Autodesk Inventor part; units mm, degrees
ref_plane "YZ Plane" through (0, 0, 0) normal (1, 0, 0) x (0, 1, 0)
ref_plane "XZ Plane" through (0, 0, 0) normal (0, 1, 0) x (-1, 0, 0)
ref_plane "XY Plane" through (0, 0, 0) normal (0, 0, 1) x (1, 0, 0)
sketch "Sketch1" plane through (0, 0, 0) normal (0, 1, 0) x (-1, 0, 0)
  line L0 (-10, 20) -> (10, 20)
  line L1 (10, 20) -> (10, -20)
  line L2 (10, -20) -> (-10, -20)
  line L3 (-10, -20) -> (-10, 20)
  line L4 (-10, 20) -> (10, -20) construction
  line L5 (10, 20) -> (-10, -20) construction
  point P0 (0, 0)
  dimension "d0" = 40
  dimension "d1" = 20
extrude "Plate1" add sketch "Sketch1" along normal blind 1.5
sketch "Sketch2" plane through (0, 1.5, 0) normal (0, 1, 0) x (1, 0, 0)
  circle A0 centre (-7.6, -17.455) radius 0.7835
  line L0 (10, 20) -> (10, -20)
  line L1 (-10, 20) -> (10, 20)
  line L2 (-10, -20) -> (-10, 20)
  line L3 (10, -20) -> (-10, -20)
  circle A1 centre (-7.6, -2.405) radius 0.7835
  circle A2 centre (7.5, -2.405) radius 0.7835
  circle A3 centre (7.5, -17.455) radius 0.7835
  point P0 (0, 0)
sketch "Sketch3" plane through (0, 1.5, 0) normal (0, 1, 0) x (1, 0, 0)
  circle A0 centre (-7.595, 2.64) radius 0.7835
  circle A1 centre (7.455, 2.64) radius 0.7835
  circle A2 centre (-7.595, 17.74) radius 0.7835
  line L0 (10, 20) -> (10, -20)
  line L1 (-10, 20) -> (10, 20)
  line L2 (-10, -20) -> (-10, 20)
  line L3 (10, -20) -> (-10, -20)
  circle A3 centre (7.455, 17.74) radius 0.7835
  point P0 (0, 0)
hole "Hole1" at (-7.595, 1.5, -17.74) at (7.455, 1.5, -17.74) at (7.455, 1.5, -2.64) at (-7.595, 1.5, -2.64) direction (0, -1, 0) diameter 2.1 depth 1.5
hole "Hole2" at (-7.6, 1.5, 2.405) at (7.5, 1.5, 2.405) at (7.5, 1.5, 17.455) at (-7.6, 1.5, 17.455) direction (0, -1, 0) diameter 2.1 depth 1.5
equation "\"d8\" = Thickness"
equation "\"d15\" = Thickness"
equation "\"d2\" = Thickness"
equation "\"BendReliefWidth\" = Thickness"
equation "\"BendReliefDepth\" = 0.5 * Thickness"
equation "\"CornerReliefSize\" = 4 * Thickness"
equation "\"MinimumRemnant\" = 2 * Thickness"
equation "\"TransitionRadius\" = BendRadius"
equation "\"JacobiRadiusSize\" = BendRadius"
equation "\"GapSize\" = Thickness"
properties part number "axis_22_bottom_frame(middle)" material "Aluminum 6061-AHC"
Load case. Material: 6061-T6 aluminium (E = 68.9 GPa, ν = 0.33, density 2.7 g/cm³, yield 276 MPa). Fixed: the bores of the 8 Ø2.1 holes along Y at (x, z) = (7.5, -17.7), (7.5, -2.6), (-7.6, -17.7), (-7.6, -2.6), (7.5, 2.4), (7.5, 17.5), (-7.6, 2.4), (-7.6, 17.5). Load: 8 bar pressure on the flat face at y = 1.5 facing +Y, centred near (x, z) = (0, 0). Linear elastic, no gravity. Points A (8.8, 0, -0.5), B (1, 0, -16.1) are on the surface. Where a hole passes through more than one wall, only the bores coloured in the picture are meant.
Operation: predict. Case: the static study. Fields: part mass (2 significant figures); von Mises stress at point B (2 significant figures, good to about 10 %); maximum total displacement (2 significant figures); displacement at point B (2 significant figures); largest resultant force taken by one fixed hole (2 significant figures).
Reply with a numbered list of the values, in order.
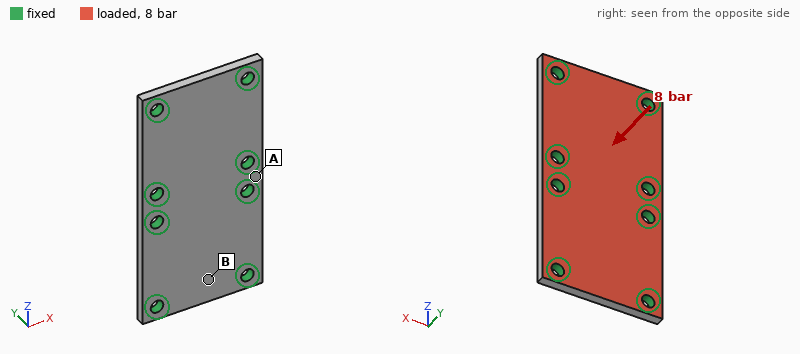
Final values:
1. 3.1 g
2. 19 MPa
3. 11 µm
4. 6.9 µm
5. 79 N
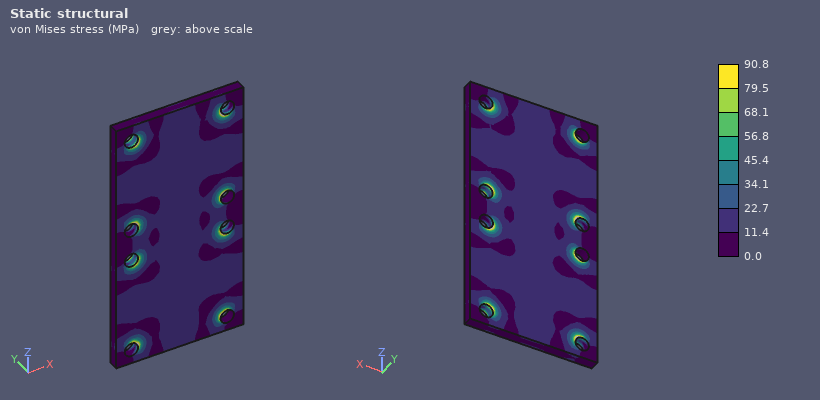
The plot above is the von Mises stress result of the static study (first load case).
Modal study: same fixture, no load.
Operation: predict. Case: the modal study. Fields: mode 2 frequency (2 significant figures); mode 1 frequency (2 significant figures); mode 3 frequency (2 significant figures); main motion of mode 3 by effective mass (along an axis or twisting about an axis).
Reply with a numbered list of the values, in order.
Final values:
1. 26 kHz
2. 26 kHz
3. 40 kHz
4. twisting about Z
